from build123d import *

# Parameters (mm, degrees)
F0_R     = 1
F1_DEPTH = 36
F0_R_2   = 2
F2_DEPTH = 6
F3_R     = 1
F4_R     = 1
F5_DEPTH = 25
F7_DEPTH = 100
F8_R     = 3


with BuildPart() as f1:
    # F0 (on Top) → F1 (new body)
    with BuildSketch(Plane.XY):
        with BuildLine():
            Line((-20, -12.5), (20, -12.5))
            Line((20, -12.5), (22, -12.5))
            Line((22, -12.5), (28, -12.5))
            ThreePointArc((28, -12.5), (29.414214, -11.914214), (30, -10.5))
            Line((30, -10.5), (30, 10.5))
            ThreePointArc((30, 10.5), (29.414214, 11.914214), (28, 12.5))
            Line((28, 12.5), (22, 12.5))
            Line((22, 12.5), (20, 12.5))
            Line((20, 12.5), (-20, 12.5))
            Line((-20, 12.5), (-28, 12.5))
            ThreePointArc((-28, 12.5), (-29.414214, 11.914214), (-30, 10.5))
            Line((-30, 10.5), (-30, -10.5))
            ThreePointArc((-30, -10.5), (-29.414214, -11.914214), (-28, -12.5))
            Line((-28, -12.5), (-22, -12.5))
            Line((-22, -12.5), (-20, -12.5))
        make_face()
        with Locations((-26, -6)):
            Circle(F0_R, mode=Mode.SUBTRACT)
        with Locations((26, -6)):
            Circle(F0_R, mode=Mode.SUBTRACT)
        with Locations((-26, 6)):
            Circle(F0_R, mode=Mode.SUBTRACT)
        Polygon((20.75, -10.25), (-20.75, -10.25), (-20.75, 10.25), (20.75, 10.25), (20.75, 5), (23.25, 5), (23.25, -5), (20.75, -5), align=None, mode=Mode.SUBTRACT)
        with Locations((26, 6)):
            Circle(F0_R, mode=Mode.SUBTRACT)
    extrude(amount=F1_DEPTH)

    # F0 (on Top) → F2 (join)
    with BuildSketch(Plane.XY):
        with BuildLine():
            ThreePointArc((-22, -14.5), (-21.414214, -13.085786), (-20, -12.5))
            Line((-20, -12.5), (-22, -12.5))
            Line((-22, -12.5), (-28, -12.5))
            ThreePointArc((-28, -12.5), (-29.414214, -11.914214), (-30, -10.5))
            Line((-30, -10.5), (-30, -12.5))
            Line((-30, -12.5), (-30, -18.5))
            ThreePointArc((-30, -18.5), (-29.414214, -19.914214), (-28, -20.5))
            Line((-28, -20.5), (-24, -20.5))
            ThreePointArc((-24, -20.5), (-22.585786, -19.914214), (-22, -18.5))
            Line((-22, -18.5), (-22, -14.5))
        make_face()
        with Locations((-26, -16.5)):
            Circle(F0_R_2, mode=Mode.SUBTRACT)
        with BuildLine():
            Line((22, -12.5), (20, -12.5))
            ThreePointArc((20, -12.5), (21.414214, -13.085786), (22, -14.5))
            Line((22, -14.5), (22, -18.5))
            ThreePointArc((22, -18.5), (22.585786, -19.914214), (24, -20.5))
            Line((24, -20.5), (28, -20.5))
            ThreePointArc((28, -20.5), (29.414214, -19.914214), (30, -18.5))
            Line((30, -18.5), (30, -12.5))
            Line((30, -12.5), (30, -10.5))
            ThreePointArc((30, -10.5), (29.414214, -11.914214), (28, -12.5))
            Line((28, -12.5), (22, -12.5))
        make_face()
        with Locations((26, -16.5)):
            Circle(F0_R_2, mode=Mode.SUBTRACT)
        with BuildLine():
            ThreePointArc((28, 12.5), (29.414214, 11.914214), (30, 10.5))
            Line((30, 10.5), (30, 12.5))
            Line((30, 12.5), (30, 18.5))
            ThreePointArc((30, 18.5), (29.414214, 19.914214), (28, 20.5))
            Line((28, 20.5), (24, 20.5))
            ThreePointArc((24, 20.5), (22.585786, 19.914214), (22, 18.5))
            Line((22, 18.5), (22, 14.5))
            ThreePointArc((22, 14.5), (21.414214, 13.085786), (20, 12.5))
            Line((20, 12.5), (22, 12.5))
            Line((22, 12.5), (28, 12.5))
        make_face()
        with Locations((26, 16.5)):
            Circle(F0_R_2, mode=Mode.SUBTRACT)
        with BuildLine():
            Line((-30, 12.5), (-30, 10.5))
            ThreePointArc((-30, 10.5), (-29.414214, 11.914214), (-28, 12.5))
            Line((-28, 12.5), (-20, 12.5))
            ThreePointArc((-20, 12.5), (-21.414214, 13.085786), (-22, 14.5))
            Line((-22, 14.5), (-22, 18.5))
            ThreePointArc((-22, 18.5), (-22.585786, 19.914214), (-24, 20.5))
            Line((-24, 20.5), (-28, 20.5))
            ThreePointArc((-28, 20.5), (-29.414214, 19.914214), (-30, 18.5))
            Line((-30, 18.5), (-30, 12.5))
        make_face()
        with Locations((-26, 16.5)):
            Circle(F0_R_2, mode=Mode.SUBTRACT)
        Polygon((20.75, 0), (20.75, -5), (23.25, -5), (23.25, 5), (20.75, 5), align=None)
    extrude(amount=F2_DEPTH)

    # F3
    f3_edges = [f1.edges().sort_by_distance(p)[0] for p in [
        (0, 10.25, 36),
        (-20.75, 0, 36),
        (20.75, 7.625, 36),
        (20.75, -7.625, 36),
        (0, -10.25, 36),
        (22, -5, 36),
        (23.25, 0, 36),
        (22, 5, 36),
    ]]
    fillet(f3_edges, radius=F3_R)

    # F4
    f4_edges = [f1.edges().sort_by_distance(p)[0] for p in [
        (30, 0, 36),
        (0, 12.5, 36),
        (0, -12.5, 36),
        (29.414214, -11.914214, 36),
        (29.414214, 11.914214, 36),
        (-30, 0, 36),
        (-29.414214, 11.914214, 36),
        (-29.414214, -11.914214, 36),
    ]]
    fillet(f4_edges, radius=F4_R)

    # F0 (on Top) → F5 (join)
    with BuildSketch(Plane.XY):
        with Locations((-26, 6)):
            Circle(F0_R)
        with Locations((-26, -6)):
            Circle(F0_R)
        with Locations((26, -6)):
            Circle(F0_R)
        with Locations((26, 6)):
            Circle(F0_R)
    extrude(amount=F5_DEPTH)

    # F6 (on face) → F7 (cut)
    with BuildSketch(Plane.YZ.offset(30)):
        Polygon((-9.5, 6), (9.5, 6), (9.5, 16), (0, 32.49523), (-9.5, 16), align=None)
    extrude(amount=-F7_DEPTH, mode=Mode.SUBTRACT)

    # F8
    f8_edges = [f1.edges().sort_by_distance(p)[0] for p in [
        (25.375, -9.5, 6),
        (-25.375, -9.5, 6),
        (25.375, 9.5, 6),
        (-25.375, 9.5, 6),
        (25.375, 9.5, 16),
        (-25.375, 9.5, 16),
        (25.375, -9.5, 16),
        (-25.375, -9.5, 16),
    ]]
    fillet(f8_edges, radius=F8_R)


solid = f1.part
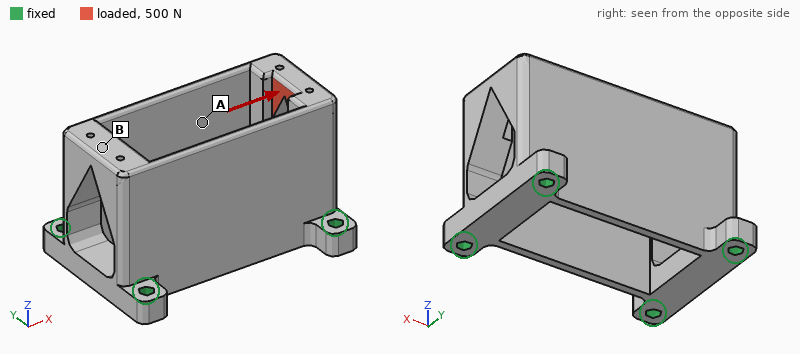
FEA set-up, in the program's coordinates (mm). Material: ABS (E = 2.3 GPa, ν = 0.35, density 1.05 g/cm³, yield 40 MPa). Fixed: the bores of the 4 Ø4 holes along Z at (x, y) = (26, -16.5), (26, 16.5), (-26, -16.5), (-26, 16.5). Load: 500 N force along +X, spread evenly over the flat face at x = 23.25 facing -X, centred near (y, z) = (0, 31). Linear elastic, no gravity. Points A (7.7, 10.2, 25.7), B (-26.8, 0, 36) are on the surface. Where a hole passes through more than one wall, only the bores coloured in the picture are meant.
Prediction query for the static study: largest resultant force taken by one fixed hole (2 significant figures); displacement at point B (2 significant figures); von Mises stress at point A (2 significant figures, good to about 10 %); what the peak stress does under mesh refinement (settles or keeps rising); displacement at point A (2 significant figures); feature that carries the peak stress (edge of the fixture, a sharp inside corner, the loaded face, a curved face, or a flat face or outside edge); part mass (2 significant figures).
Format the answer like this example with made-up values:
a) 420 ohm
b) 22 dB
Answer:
a) 200 N
b) 0.093 mm
c) 8.5 MPa
d) keeps rising
e) 0.34 mm
f) a sharp inside corner
g) 19 g
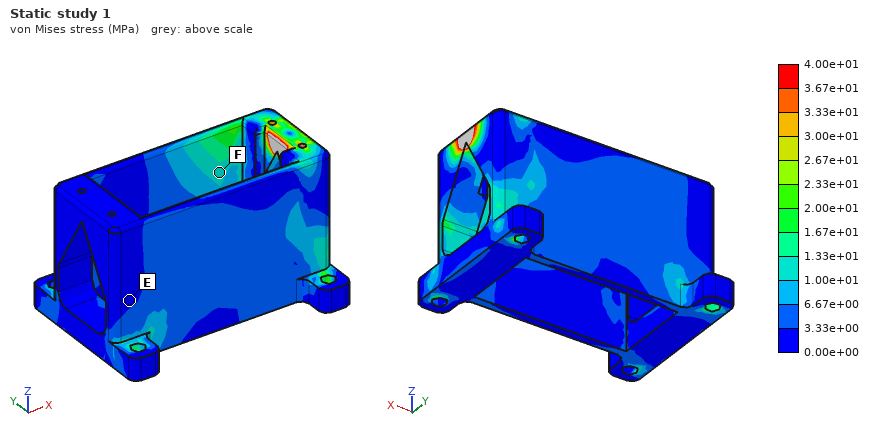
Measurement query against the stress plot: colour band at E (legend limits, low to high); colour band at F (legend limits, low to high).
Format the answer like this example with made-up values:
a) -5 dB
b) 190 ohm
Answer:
a) 0.00e+00 to 3.33e+00 MPa
b) 1.00e+01 to 1.33e+01 MPa
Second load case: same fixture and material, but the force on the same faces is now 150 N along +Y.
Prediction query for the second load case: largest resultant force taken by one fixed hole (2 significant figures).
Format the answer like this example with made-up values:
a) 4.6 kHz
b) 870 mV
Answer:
a) 150 N
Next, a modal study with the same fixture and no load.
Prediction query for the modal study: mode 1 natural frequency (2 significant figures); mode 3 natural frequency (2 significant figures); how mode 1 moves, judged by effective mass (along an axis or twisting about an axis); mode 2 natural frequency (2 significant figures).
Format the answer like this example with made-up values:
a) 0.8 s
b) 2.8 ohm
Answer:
a) 1300 Hz
b) 1600 Hz
c) along Y
d) 1600 Hz
